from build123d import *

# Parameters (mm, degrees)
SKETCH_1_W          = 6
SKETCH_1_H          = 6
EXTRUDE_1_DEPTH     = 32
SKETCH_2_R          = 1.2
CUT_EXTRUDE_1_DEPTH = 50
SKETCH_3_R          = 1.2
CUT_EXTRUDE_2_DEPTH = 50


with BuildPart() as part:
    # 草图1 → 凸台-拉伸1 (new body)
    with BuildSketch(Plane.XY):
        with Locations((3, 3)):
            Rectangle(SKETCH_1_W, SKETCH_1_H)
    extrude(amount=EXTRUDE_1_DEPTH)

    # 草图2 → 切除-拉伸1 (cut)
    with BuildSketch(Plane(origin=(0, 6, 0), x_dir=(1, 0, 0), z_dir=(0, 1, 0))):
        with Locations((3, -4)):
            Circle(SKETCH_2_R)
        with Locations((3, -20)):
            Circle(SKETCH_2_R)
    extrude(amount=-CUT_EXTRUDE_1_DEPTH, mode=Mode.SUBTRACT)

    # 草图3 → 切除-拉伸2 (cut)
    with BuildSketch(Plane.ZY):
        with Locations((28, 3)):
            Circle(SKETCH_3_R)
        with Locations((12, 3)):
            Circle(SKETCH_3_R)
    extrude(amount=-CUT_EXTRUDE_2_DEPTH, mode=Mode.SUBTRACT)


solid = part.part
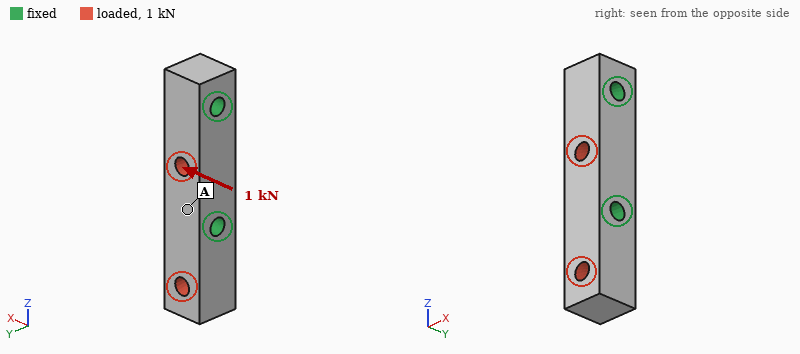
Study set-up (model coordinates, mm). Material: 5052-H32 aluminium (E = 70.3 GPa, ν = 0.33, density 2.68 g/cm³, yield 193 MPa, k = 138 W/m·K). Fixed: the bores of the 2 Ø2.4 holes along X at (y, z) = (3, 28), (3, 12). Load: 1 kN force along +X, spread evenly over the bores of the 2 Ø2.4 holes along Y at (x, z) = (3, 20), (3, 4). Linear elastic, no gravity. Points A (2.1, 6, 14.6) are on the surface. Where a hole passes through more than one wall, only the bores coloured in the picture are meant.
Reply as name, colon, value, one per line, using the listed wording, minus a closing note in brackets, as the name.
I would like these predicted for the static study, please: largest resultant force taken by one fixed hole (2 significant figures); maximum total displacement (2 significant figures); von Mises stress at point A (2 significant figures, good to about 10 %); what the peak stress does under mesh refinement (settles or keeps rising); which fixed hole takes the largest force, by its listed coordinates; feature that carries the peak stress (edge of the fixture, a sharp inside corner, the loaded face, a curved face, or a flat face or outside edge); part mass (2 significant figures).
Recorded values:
largest resultant force taken by one fixed hole: 770 N
maximum total displacement: 24 µm
von Mises stress at point A: 19 MPa
what the peak stress does under mesh refinement: keeps rising
which fixed hole takes the largest force, by its listed coordinates: (3, 12)
feature that carries the peak stress: edge of the fixture
part mass: 2.8 g
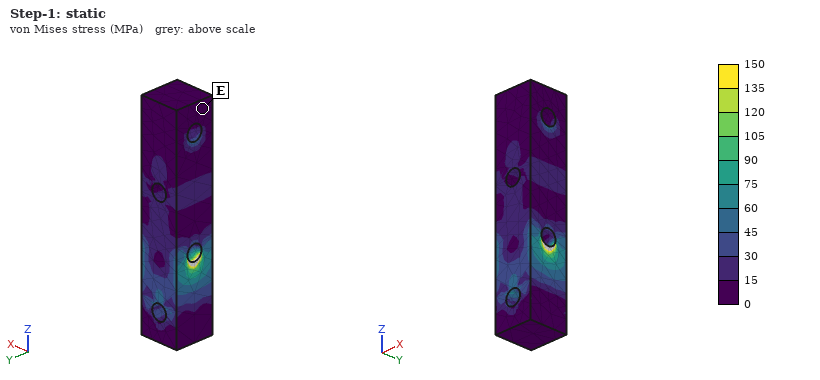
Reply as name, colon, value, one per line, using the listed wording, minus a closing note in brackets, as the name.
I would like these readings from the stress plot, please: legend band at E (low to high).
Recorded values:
legend band at E: 0 to 15 MPa
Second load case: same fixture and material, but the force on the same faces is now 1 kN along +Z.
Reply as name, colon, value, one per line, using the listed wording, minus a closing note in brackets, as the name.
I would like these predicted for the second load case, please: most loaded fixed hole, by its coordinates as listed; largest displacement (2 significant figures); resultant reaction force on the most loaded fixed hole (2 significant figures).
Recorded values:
most loaded fixed hole, by its coordinates as listed: (3, 12)
largest displacement: 2.3 µm
resultant reaction force on the most loaded fixed hole: 740 N
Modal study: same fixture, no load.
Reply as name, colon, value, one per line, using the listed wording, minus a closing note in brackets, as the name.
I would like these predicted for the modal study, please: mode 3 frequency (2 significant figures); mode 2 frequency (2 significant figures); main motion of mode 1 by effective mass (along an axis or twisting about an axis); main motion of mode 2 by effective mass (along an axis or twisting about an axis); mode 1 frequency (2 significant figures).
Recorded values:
mode 3 frequency: 61 kHz
mode 2 frequency: 31 kHz
main motion of mode 1 by effective mass: along Y
main motion of mode 2 by effective mass: along X
mode 1 frequency: 27 kHz
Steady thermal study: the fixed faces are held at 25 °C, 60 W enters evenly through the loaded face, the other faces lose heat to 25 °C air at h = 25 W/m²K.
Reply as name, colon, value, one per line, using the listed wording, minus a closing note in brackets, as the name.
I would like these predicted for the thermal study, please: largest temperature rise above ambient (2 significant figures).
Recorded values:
largest temperature rise above ambient: 54 K
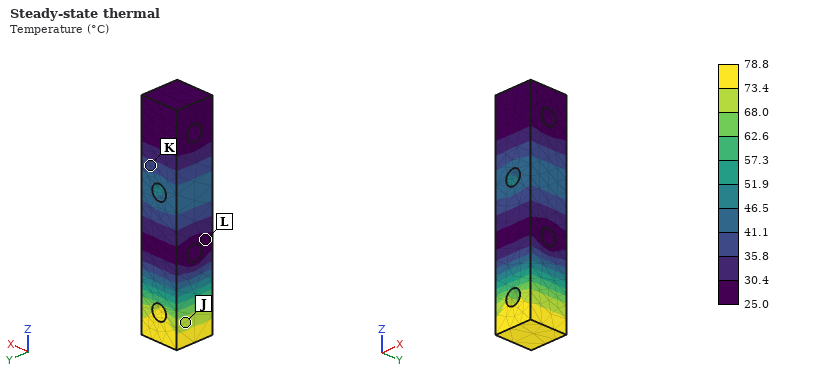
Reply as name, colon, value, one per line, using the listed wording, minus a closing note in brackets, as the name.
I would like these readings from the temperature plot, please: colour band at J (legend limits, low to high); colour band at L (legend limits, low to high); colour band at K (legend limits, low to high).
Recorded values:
colour band at J: 68.0 to 73.4 °C
colour band at L: 25.0 to 30.4 °C
colour band at K: 35.8 to 41.1 °C
